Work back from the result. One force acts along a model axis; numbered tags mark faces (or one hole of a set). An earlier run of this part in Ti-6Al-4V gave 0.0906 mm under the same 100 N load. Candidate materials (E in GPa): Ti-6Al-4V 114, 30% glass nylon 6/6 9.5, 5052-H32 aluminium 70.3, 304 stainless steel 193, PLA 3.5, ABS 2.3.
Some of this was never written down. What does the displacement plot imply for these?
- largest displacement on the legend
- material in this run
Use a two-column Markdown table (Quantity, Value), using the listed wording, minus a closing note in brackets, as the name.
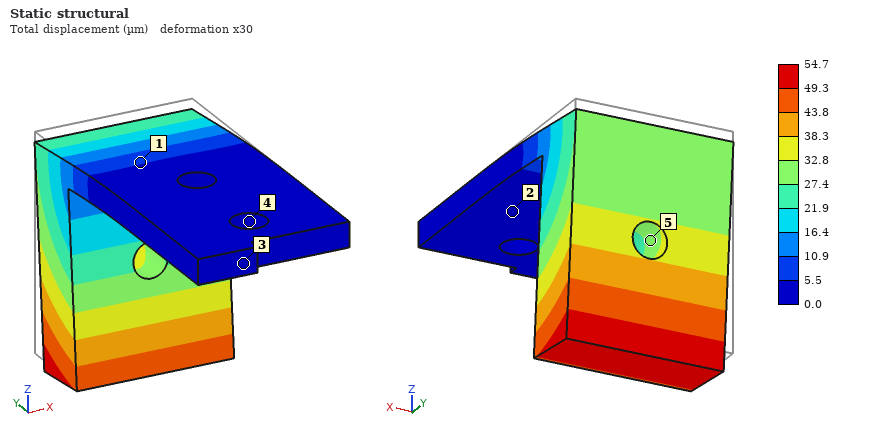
| Quantity | Value |
|---|---|
| largest displacement on the legend | 54.7 µm |
| material in this run | 304 stainless steel |
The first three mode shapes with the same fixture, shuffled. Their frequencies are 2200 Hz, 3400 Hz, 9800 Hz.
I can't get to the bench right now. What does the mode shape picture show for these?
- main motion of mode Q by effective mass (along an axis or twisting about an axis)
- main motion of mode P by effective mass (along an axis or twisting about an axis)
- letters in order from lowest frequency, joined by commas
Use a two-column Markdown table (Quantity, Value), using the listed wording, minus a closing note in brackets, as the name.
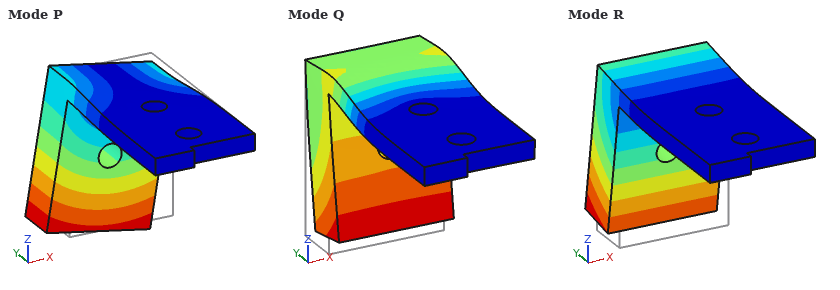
| Quantity | Value |
|---|---|
| main motion of mode Q by effective mass | along Z |
| main motion of mode P by effective mass | along X |
| letters in order from lowest frequency, joined by commas | R, P, Q |
